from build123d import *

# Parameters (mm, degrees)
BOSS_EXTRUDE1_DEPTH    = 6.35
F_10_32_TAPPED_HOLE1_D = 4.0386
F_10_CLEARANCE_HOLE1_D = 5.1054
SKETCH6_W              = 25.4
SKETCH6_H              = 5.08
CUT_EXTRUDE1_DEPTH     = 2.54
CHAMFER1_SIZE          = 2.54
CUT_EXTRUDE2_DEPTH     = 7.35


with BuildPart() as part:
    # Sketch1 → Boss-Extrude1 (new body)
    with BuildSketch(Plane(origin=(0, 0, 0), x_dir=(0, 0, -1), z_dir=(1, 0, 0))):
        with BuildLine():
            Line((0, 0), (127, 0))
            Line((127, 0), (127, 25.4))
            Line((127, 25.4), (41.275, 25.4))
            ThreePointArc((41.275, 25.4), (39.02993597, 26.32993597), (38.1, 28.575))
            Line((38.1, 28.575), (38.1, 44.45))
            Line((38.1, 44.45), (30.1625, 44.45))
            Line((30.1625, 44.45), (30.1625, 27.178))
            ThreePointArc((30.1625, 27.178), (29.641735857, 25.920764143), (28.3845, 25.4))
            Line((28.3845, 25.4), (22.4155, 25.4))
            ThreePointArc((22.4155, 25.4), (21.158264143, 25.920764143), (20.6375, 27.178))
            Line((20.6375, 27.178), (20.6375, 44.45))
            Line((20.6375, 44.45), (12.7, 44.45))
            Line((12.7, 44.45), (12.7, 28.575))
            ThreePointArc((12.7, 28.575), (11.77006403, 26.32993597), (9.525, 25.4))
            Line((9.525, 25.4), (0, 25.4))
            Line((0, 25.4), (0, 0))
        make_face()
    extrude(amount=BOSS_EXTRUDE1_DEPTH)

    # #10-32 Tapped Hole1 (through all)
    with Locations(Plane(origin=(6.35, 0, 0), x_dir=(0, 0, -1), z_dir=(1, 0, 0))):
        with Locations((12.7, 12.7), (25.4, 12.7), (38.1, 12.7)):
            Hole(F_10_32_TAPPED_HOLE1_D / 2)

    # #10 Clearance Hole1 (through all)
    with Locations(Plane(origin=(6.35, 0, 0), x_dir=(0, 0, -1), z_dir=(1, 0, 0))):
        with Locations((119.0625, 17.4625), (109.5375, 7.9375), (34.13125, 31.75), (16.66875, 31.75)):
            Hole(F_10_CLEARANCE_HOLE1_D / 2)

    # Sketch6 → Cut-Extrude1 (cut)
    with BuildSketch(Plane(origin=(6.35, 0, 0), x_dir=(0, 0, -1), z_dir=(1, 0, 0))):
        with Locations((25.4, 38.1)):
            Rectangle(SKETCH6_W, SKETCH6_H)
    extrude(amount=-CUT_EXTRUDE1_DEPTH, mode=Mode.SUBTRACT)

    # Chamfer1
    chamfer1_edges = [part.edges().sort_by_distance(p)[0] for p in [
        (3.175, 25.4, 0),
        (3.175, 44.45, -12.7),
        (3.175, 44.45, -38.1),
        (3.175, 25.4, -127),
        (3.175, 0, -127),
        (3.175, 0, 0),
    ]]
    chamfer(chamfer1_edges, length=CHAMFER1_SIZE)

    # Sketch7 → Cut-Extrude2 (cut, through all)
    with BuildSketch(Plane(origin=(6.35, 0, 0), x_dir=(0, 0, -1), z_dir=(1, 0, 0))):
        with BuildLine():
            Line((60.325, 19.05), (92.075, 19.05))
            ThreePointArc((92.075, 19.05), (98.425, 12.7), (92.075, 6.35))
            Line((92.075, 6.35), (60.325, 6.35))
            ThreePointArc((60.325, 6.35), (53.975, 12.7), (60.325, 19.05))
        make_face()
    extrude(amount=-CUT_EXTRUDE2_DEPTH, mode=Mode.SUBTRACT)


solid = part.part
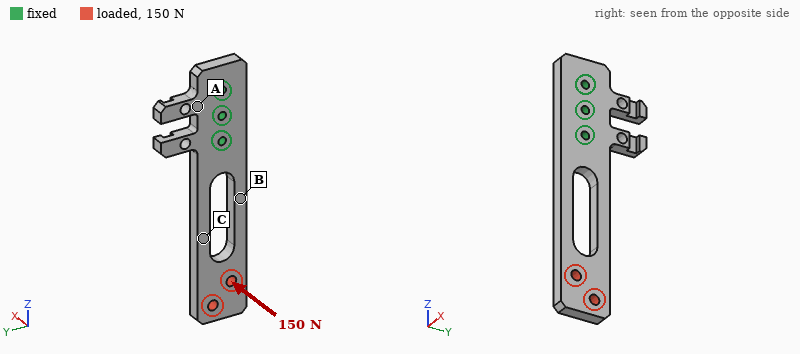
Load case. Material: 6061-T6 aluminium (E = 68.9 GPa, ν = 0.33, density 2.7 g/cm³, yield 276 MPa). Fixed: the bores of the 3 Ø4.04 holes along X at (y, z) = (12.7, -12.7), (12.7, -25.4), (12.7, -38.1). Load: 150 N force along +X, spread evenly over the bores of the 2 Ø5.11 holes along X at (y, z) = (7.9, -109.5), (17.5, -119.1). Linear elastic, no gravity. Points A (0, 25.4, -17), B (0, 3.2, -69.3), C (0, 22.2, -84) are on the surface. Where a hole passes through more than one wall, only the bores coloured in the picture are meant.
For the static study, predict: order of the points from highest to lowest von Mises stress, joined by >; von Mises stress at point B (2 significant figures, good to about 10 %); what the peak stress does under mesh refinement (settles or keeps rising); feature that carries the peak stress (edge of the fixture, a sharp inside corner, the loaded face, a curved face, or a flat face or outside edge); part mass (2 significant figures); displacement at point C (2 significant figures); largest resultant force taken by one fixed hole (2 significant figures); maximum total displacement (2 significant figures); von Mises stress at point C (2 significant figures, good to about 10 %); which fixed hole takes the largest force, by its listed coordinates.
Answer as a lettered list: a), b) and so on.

a) B > C > A
b) 79 MPa
c) keeps rising
d) edge of the fixture
e) 49 g
f) 0.36 mm
g) 500 N
h) 1.1 mm
i) 53 MPa
j) (12.7, -38.1)
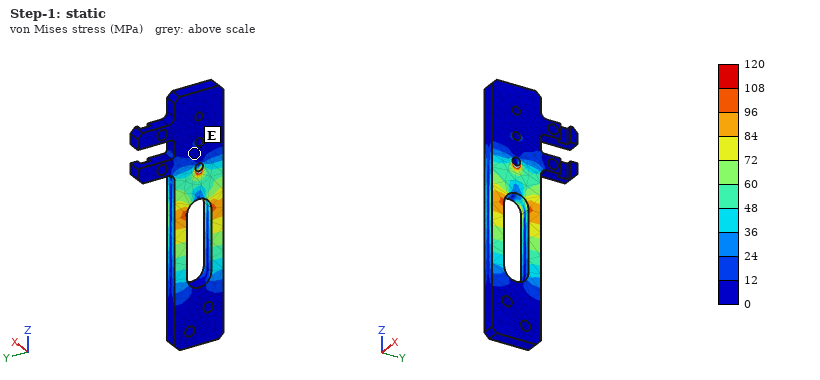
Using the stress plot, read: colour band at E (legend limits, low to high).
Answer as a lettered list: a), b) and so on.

a) 0 to 12 MPa
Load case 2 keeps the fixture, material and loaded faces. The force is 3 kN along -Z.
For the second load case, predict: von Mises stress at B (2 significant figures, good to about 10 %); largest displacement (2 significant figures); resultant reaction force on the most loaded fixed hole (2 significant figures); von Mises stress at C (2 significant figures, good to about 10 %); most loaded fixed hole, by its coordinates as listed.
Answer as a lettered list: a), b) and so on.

a) 37 MPa
b) 40 µm
c) 2.0 kN
d) 37 MPa
e) (12.7, -38.1)
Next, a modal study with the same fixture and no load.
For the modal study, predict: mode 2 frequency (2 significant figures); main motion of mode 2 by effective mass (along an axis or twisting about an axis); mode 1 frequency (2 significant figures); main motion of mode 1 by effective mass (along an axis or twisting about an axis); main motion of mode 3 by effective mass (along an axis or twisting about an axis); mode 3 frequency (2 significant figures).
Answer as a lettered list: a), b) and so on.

a) 1500 Hz
b) along Y
c) 580 Hz
d) along X
e) twisting about Z
f) 2800 Hz
